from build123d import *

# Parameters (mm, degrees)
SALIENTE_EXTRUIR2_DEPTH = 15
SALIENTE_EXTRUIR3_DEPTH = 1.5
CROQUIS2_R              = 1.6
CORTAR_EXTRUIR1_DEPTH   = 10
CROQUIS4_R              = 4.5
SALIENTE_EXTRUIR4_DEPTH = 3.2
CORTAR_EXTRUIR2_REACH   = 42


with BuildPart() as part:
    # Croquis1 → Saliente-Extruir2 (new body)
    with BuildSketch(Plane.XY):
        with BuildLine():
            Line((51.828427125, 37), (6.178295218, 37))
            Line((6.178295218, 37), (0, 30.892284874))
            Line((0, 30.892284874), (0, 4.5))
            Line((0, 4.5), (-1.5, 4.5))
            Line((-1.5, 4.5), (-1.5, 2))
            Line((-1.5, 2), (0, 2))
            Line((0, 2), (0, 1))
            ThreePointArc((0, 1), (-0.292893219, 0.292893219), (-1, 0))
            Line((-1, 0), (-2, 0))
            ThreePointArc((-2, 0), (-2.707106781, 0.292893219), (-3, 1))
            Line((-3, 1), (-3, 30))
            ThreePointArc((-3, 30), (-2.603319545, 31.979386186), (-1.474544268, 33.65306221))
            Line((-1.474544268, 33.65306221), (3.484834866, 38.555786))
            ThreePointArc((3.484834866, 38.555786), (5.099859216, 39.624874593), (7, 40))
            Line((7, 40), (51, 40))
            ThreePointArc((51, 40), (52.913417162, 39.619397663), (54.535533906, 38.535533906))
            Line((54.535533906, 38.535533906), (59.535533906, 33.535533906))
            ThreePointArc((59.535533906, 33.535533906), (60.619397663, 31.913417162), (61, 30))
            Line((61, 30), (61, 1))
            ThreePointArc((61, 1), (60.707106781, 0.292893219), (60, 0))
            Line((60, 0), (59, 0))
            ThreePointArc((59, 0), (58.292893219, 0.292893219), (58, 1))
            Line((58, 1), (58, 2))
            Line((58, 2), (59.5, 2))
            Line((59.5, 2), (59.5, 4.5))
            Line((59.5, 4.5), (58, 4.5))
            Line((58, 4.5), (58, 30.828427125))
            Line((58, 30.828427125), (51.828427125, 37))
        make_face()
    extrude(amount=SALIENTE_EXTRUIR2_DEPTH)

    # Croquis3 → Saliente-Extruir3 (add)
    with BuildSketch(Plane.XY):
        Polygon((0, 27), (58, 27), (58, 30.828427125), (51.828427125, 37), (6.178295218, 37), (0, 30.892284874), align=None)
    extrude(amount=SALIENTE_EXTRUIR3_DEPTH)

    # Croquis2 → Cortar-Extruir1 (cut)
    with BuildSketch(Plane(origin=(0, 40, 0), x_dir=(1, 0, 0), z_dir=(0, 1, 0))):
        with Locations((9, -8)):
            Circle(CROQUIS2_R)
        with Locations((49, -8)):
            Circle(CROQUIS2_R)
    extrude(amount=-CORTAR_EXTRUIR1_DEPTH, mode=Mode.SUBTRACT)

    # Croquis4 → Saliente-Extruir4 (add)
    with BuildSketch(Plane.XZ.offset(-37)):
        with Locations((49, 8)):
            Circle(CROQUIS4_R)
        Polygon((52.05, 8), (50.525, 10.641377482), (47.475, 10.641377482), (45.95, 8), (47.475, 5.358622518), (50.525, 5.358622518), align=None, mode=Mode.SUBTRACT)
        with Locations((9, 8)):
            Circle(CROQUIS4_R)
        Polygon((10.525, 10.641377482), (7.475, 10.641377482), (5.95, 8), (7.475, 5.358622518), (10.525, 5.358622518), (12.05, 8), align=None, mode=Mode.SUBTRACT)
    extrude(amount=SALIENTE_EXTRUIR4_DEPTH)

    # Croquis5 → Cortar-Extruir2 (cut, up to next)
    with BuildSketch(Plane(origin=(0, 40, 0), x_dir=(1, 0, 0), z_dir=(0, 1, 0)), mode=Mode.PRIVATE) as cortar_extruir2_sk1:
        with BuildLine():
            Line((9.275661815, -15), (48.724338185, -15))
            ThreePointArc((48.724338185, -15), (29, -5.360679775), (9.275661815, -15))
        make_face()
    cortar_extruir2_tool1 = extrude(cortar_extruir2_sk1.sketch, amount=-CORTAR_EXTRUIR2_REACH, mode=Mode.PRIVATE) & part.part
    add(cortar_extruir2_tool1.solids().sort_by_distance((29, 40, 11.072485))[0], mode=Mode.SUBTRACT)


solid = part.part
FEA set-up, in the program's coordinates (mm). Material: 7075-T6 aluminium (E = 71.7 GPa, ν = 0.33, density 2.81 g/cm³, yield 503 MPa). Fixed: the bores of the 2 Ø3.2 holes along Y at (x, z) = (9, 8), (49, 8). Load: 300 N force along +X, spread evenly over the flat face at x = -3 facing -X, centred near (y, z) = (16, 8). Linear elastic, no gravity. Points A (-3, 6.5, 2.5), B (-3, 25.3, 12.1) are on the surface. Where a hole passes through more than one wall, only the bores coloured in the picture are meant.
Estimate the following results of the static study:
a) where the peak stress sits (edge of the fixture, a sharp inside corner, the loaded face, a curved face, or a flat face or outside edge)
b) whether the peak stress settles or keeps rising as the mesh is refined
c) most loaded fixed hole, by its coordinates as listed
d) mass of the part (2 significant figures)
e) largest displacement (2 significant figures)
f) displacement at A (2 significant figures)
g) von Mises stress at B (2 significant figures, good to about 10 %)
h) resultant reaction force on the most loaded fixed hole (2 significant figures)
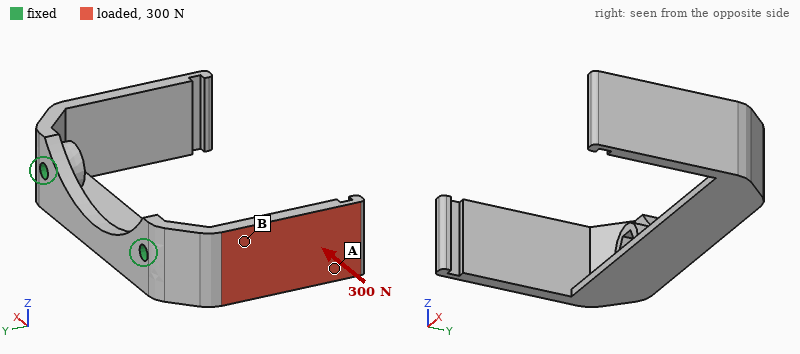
a sharp inside corner
keeps rising
(9, 8)
17 g
0.82 mm
0.54 mm
110 MPa
210 N
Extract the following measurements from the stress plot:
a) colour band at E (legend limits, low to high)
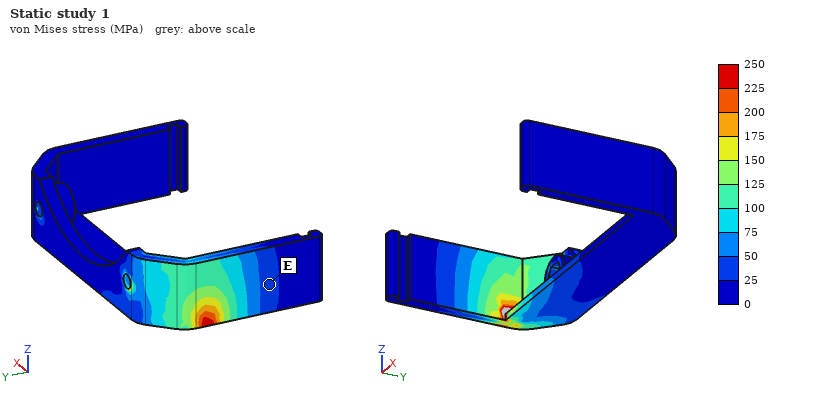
25 to 50 MPa
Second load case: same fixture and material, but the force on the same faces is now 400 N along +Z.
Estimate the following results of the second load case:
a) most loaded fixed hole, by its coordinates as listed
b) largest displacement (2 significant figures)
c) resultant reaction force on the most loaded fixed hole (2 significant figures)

(9, 8)
0.49 mm
450 N
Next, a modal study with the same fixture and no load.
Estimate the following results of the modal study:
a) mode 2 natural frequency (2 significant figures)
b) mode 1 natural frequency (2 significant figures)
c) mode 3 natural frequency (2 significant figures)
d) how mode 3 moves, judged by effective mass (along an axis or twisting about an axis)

2100 Hz
2100 Hz
2800 Hz
twisting about Y
